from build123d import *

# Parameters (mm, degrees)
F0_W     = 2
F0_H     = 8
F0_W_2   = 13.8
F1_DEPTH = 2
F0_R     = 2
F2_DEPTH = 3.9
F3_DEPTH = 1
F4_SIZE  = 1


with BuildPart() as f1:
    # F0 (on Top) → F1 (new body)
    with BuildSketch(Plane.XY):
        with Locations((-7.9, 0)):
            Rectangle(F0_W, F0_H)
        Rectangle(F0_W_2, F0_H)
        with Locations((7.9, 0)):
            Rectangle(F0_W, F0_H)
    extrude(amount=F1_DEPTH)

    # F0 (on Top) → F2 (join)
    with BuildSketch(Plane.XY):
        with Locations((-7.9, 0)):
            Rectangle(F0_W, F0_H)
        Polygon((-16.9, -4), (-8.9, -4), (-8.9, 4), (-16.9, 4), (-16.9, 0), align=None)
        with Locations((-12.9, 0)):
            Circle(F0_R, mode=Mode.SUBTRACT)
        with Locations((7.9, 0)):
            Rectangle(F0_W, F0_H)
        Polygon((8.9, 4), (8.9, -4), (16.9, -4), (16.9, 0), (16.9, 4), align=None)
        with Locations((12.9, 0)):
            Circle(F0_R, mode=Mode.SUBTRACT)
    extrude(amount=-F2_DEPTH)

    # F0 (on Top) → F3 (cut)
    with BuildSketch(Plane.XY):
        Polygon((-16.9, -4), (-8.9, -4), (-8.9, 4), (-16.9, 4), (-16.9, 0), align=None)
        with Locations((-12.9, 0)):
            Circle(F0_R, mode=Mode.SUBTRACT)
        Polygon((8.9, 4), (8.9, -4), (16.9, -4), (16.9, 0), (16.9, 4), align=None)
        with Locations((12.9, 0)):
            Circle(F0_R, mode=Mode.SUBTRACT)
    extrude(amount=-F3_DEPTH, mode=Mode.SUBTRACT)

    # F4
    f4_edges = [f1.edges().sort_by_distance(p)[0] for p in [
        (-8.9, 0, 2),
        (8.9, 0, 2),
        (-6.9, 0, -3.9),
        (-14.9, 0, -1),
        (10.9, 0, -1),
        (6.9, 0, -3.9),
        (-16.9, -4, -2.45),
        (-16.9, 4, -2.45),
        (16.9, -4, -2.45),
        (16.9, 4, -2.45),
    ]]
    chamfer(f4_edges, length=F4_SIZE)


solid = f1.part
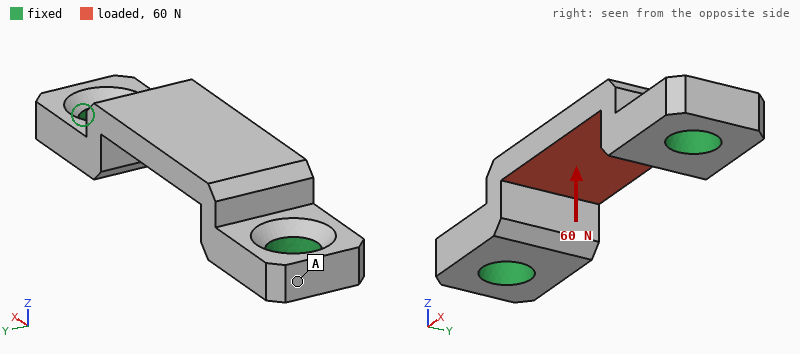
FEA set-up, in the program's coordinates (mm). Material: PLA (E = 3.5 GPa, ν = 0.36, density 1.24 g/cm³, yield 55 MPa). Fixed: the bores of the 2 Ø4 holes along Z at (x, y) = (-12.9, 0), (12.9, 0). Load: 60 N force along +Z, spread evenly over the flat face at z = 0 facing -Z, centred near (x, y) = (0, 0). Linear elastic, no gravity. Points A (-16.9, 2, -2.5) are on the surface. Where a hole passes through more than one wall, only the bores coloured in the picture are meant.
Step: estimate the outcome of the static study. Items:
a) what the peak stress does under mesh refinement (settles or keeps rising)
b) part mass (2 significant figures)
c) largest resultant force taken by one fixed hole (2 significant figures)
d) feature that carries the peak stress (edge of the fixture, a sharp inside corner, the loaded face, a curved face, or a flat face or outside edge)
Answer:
keeps rising
0.83 g
49 N
edge of the fixture
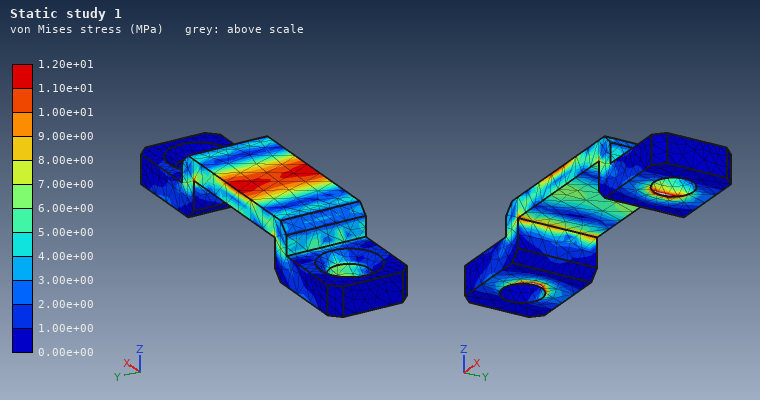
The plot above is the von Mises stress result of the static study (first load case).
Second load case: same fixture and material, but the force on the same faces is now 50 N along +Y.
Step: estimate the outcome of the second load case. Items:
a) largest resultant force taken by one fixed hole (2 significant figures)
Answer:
25 N
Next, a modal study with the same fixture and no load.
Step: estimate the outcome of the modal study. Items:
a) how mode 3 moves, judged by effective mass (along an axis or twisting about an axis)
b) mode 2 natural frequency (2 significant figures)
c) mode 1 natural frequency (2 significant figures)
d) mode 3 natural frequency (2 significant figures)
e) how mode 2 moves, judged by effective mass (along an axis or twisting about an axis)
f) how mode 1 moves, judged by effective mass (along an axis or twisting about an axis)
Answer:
along X
11 kHz
9400 Hz
11 kHz
along Z
along Y
